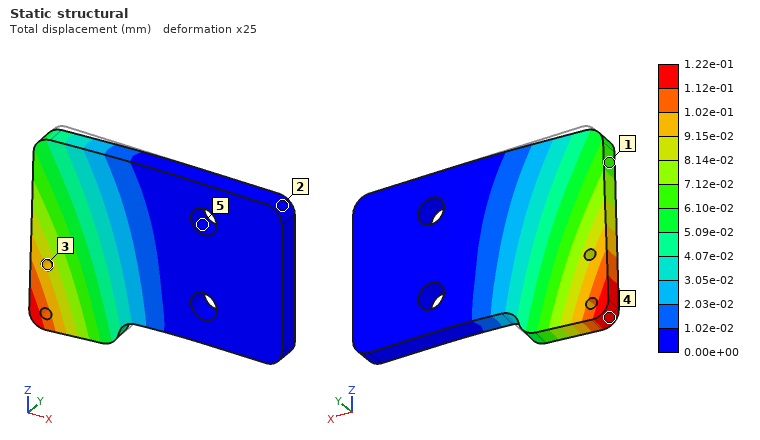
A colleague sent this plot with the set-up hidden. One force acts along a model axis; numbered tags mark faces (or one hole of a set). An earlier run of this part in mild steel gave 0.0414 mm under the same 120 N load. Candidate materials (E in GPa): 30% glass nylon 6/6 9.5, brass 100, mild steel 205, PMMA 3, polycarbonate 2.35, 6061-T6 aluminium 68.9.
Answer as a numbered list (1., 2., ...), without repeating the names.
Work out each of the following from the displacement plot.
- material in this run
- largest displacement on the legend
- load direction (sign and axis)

1. 6061-T6 aluminium
2. 1.22e-01 mm
3. -Y
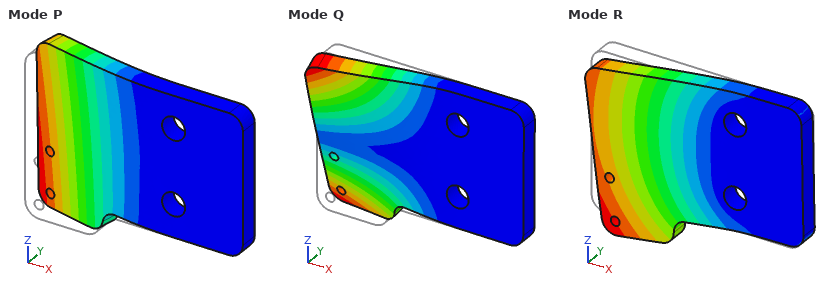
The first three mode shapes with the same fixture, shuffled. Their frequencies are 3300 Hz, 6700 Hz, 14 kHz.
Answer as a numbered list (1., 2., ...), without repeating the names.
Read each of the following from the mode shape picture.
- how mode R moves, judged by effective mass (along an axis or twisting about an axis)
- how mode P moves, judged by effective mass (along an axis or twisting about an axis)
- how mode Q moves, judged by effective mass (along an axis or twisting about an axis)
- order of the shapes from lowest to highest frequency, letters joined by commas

1. along Z
2. along Y
3. twisting about X
4. P, Q, R
